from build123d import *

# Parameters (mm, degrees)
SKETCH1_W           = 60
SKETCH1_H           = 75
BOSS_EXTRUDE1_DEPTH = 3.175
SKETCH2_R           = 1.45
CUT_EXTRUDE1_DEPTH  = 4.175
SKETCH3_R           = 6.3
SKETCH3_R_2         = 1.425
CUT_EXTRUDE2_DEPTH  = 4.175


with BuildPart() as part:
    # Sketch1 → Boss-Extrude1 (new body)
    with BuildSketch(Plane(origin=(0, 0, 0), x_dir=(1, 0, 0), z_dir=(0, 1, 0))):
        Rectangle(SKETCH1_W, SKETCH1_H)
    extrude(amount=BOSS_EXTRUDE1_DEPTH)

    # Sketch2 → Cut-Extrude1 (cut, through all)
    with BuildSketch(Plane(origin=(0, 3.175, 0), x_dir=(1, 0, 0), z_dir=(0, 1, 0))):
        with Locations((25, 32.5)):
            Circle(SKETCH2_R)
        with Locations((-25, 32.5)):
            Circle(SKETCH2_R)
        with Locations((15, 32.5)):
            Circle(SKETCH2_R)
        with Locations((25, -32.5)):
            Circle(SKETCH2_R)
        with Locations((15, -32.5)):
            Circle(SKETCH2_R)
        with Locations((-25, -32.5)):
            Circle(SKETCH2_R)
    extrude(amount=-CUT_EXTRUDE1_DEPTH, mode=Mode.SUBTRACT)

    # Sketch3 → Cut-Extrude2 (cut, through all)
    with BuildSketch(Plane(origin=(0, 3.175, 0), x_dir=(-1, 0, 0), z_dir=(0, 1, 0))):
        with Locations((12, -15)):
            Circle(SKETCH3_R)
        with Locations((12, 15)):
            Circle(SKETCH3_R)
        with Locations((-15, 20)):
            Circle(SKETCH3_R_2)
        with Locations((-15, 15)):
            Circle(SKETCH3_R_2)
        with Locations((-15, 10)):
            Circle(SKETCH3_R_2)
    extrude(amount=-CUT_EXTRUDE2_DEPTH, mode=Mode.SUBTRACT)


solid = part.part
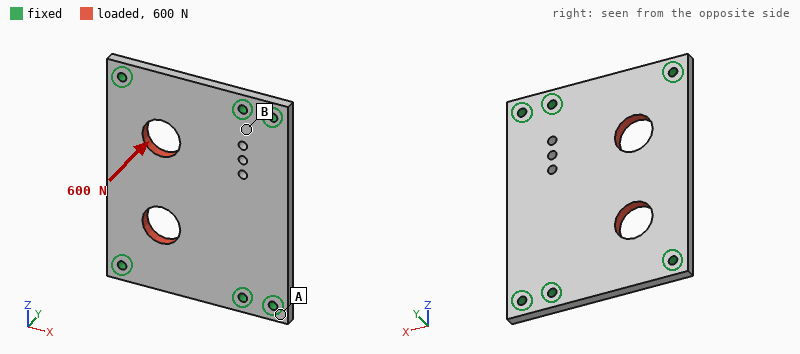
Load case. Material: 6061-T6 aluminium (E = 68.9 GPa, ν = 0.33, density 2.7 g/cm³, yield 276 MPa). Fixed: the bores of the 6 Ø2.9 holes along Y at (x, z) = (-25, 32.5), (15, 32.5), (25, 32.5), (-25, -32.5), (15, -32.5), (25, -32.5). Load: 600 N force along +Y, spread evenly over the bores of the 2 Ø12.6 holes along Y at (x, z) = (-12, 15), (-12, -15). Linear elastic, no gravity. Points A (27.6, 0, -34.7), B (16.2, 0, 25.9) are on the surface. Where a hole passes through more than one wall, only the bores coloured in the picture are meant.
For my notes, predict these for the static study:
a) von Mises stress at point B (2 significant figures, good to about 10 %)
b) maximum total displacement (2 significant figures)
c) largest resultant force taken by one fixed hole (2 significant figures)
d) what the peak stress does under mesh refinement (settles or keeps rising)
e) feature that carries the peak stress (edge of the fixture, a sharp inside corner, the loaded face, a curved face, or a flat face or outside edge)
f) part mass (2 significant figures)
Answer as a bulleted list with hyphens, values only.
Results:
- 25 MPa
- 0.10 mm
- 210 N
- keeps rising
- edge of the fixture
- 36 g
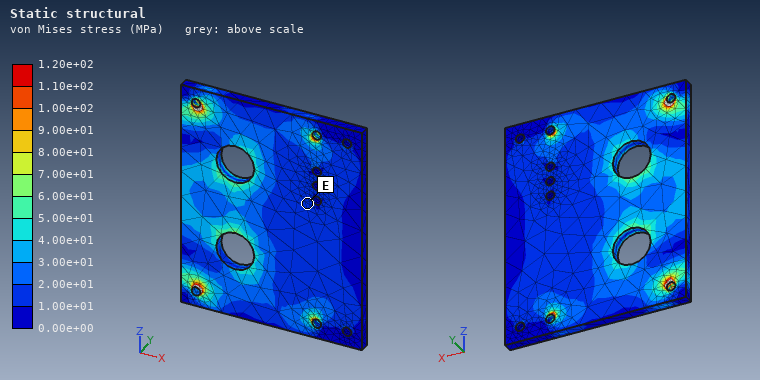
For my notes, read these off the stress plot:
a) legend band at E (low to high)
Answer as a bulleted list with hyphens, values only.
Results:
- 1.00e+01 to 2.00e+01 MPa
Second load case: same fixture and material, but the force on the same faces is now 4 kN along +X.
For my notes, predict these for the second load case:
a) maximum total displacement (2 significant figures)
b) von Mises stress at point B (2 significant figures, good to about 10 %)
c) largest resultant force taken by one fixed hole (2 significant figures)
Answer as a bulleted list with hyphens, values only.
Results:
- 17 µm
- 22 MPa
- 960 N
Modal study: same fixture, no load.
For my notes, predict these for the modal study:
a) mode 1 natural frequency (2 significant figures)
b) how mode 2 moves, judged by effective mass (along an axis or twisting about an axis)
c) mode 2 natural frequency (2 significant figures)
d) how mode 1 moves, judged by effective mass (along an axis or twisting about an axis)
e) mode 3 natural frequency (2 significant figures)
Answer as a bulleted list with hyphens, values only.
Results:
- 3400 Hz
- twisting about Z
- 4700 Hz
- along Y
- 7100 Hz
